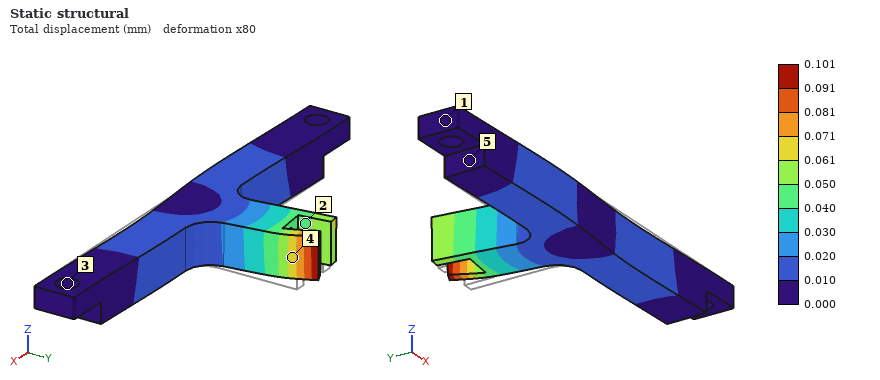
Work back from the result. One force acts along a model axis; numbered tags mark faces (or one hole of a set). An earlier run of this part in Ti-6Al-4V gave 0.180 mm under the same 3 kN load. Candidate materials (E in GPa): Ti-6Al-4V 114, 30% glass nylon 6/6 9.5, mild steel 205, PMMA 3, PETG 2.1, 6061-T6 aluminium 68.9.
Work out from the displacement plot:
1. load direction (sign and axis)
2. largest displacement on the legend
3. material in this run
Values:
-X
0.101 mm
mild steel
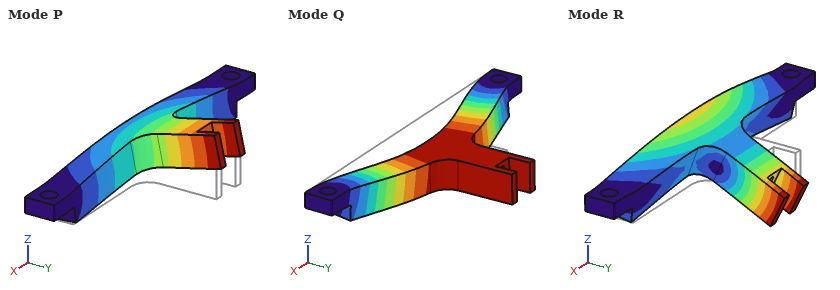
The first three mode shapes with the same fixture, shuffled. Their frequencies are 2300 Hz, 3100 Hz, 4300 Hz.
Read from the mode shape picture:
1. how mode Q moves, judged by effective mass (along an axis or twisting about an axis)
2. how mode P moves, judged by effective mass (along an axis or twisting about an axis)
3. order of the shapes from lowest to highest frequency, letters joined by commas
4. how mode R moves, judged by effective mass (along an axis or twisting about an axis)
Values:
along Y
along Z
P, Q, R
along Z
